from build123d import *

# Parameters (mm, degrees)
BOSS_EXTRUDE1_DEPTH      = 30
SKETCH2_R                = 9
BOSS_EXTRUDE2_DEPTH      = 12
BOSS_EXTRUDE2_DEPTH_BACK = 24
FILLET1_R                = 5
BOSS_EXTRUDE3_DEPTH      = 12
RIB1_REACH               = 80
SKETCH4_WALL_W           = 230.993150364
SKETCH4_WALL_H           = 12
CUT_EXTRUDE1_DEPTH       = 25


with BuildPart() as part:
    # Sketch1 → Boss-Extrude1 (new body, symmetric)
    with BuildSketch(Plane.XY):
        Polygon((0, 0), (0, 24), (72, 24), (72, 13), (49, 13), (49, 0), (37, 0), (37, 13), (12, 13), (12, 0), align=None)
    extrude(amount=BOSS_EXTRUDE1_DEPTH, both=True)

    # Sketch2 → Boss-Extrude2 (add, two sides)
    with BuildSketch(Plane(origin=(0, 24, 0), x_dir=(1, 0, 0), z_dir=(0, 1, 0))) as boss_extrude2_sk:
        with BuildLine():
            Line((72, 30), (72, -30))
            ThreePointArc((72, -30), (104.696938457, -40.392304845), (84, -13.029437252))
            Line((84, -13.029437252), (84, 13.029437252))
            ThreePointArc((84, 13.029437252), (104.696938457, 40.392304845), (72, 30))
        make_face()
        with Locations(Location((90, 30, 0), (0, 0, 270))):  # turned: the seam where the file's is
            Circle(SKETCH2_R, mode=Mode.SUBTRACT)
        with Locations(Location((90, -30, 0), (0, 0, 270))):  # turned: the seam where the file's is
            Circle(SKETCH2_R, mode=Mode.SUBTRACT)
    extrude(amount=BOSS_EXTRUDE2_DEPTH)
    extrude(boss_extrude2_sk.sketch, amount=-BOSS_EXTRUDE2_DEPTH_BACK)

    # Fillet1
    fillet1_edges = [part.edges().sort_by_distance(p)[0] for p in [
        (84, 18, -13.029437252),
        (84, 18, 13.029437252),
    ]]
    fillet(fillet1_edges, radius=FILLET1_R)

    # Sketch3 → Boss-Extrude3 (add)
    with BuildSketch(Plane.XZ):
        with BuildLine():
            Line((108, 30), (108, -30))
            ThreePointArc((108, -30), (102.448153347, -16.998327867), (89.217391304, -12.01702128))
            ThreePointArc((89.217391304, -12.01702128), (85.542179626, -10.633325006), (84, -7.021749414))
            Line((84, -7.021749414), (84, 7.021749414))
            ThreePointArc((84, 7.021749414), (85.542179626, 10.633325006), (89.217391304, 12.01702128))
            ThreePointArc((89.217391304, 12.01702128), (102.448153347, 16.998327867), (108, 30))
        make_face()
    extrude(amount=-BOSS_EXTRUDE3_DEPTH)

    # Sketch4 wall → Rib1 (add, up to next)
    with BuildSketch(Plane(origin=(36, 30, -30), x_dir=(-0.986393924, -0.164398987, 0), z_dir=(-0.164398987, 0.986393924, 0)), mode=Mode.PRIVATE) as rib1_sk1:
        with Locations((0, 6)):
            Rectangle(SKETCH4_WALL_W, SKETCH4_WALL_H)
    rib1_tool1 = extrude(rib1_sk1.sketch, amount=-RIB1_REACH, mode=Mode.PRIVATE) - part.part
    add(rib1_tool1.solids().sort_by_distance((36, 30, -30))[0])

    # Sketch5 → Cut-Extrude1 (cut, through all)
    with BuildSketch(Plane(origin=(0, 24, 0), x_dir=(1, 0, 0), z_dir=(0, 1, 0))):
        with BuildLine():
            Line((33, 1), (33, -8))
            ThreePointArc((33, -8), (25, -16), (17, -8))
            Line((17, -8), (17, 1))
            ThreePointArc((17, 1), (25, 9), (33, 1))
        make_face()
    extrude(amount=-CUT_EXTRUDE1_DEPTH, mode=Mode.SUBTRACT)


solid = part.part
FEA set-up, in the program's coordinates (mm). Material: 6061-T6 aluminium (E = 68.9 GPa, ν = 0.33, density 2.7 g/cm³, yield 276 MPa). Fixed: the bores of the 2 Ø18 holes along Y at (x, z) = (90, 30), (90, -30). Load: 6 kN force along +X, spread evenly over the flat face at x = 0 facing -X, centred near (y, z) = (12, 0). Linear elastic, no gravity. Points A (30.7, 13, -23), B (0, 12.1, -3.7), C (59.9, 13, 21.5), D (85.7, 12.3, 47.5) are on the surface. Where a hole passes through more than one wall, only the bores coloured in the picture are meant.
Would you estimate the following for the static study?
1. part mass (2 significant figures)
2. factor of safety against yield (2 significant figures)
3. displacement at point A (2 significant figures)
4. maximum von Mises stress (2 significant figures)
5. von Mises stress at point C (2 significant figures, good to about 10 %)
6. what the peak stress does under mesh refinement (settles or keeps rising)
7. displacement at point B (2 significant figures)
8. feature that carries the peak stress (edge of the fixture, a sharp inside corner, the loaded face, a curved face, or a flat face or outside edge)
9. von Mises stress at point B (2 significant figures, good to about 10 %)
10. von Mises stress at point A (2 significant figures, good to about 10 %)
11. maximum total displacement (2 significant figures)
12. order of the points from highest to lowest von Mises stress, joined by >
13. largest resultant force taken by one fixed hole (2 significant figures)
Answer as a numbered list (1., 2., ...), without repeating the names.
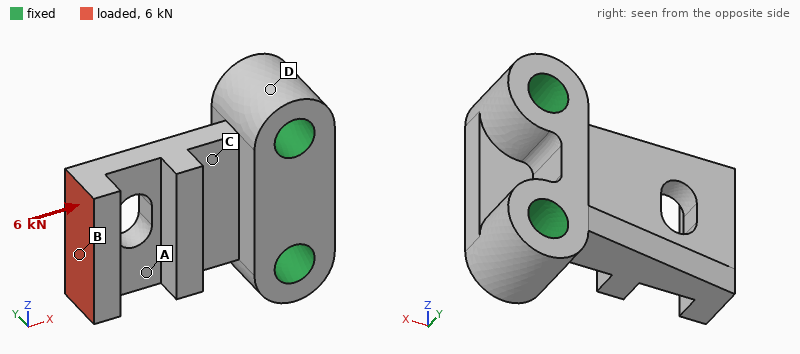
1. 400 g
2. 2.6
3. 0.049 mm
4. 110 MPa
5. 29 MPa
6. settles
7. 0.17 mm
8. a curved face
9. 14 MPa
10. 48 MPa
11. 0.20 mm
12. A > C > B > D
13. 3.2 kN
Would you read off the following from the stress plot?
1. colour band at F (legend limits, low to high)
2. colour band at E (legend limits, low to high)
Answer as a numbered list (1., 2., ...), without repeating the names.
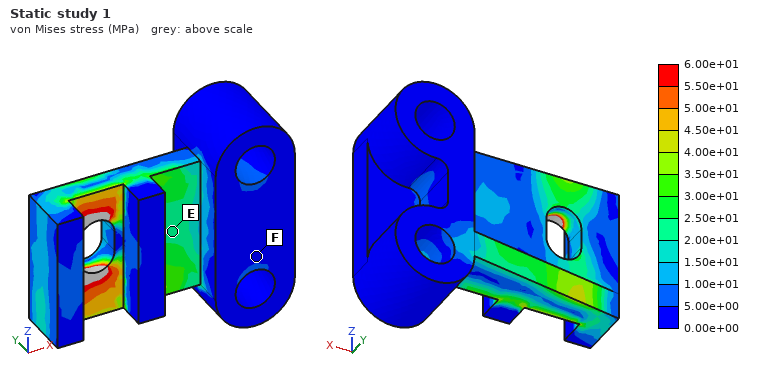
1. 0.00e+00 to 5.00e+00 MPa
2. 2.00e+01 to 2.50e+01 MPa
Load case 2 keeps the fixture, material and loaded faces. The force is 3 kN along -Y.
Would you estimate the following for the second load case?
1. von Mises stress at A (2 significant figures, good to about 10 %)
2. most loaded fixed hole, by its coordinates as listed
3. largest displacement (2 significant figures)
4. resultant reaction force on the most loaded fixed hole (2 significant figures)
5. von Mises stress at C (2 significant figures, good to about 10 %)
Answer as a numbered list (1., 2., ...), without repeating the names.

1. 87 MPa
2. (90, -30)
3. 0.61 mm
4. 1.7 kN
5. 73 MPa
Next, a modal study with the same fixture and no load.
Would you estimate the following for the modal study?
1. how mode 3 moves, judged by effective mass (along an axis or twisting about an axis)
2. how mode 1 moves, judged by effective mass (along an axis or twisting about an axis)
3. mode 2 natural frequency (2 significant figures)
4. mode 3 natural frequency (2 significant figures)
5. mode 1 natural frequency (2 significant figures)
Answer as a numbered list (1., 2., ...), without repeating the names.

1. along Z
2. along Y
3. 4000 Hz
4. 5000 Hz
5. 1700 Hz
